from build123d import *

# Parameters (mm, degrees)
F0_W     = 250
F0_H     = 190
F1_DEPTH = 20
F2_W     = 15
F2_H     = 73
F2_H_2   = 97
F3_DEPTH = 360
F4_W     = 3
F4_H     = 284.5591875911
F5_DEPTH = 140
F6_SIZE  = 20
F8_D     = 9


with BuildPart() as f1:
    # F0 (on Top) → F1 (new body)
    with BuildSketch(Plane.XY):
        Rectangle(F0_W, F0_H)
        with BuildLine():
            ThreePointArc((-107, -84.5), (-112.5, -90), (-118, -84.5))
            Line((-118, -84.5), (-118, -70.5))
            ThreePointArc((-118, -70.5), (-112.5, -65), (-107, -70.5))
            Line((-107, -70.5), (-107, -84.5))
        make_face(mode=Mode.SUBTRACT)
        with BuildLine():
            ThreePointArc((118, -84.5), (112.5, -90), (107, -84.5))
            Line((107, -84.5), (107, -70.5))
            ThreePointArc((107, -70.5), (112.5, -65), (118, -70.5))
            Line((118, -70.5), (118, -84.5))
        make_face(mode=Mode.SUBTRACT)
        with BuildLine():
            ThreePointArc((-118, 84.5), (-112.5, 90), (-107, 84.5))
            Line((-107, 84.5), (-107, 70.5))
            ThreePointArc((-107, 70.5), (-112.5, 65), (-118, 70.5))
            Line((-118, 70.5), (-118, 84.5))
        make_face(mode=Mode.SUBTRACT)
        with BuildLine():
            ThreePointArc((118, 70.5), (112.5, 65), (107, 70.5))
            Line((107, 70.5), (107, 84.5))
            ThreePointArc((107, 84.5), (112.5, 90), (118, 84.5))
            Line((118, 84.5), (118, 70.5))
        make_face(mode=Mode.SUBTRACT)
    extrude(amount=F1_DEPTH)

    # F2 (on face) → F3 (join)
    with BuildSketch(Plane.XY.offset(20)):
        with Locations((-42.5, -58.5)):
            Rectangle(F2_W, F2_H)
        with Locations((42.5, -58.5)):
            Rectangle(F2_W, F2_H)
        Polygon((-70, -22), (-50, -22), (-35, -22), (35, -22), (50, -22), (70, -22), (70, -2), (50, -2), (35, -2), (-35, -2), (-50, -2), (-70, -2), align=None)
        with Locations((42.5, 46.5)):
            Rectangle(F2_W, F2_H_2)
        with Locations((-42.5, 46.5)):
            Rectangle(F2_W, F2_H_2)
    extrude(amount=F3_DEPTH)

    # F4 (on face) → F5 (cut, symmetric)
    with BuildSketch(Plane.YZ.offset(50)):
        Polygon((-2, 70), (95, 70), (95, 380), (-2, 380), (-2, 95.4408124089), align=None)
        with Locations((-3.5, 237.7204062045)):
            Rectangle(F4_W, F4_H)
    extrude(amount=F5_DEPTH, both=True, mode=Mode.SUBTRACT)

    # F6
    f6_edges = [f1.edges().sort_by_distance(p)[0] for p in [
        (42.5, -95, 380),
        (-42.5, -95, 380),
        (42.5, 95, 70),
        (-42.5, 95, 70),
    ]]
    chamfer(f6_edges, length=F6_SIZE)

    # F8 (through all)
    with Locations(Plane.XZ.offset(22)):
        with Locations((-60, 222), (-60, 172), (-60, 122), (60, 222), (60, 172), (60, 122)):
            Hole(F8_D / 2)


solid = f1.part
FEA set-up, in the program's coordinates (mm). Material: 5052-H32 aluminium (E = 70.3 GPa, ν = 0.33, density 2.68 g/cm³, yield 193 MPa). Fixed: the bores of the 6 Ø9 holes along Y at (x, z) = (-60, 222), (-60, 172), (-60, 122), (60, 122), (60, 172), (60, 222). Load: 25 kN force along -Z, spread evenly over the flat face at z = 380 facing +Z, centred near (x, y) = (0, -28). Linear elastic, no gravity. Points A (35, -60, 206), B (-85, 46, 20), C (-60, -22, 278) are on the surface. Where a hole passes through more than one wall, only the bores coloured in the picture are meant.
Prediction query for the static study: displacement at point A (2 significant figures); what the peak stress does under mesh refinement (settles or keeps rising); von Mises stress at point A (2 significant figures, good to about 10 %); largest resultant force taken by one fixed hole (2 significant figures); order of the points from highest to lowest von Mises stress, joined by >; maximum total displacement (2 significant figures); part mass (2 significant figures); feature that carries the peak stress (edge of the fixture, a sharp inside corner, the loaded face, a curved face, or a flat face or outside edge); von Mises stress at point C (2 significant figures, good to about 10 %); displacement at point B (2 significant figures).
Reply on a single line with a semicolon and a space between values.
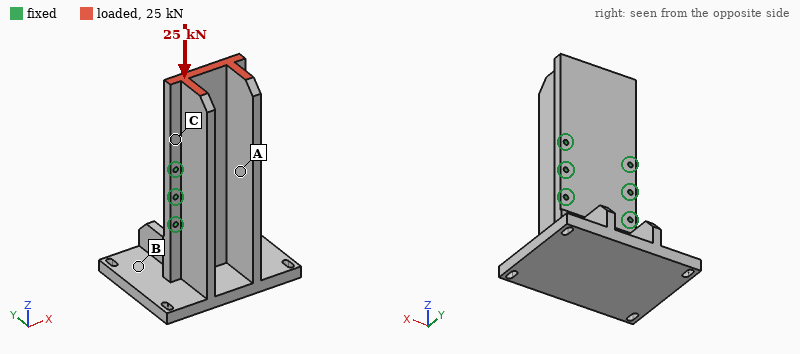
8.8 µm; keeps rising; 3.7 MPa; 7.4 kN; C > A > B; 23 µm; 7.3 kg; edge of the fixture; 6.8 MPa; 14 µm
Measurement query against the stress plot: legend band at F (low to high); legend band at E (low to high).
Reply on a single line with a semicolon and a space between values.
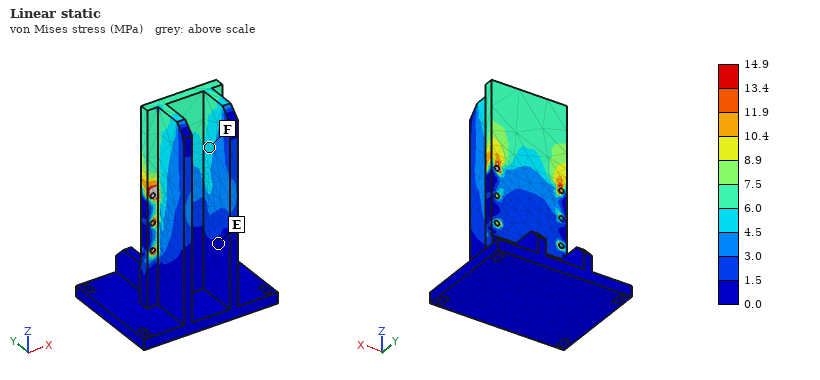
4.5 to 6.0 MPa; 0.0 to 1.5 MPa
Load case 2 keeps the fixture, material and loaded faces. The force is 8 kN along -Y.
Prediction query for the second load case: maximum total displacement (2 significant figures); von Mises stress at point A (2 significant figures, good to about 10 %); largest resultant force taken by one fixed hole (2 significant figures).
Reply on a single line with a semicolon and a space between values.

0.19 mm; 11 MPa; 10 kN
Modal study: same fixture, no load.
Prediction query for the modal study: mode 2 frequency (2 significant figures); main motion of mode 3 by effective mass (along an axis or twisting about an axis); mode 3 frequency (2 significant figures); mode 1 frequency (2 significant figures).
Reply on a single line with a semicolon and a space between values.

740 Hz; along X; 1400 Hz; 730 Hz
